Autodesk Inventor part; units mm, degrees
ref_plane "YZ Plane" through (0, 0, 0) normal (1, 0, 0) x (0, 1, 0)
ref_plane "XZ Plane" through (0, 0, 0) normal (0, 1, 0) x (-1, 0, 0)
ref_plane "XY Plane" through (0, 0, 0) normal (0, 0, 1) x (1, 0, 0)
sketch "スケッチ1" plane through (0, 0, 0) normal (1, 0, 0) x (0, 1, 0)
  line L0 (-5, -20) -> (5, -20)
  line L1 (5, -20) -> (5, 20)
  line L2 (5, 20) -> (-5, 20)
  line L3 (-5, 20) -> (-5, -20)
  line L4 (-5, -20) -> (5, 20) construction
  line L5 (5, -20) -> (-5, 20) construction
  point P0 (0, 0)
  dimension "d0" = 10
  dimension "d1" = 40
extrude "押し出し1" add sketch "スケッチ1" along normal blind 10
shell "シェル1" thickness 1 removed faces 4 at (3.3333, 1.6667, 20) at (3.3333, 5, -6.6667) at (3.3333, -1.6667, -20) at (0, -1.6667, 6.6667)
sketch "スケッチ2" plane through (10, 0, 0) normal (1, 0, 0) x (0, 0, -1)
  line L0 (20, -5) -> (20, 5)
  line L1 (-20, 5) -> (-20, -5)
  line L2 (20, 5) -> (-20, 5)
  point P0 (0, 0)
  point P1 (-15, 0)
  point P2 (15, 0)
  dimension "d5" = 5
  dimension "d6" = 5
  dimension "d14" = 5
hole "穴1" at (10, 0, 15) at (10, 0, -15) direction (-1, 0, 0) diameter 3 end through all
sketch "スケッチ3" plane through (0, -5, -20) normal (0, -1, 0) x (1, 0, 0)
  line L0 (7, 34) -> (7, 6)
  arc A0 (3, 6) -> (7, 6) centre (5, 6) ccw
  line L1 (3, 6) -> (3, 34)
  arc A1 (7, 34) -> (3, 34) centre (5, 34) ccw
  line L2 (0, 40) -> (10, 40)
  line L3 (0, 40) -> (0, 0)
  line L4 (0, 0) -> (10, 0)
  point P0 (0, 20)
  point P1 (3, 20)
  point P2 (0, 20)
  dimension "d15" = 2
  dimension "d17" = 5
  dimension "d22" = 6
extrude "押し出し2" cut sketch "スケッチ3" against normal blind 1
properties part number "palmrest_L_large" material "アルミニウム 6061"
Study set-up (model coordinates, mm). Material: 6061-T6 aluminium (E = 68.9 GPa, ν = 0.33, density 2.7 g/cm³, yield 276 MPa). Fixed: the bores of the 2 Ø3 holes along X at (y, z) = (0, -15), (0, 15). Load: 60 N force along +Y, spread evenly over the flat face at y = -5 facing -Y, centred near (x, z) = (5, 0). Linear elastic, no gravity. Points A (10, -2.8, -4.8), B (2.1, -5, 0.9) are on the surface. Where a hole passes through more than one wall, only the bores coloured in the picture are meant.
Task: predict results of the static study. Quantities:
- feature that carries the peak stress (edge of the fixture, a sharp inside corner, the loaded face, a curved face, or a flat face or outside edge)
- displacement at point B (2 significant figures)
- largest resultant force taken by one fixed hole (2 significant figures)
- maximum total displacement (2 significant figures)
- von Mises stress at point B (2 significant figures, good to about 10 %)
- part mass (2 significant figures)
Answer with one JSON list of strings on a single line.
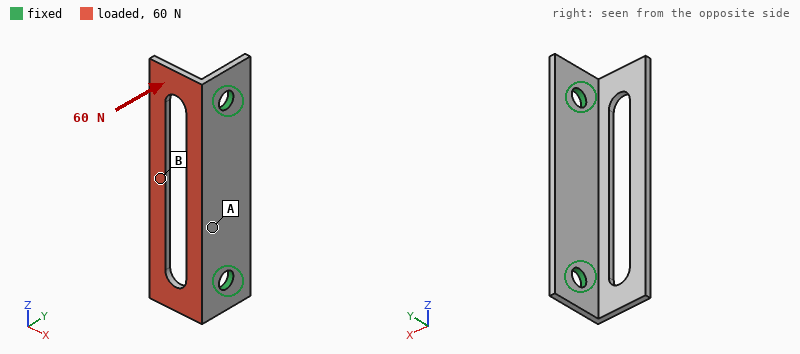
["a curved face", "0.33 mm", "30 N", "0.38 mm", "80 MPa", "1.7 g"]
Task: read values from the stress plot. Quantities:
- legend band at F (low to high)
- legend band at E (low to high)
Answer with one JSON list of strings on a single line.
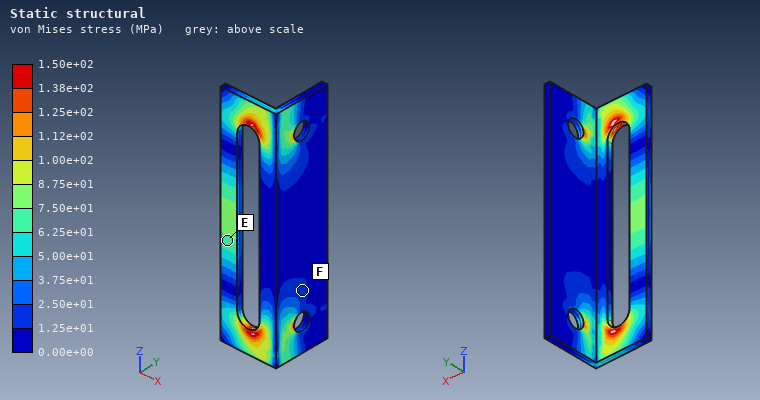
["1.25e+01 to 2.50e+01 MPa", "6.25e+01 to 7.50e+01 MPa"]
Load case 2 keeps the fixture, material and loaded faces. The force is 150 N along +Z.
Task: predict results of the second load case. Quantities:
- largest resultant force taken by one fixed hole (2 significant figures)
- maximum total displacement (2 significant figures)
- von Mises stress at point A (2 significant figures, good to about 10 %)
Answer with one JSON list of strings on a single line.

["81 N", "43 µm", "13 MPa"]
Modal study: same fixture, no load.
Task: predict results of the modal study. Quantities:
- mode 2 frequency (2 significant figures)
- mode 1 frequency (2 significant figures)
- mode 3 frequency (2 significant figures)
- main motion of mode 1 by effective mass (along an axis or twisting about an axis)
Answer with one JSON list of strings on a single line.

["5700 Hz", "2800 Hz", "7100 Hz", "along Y"]
